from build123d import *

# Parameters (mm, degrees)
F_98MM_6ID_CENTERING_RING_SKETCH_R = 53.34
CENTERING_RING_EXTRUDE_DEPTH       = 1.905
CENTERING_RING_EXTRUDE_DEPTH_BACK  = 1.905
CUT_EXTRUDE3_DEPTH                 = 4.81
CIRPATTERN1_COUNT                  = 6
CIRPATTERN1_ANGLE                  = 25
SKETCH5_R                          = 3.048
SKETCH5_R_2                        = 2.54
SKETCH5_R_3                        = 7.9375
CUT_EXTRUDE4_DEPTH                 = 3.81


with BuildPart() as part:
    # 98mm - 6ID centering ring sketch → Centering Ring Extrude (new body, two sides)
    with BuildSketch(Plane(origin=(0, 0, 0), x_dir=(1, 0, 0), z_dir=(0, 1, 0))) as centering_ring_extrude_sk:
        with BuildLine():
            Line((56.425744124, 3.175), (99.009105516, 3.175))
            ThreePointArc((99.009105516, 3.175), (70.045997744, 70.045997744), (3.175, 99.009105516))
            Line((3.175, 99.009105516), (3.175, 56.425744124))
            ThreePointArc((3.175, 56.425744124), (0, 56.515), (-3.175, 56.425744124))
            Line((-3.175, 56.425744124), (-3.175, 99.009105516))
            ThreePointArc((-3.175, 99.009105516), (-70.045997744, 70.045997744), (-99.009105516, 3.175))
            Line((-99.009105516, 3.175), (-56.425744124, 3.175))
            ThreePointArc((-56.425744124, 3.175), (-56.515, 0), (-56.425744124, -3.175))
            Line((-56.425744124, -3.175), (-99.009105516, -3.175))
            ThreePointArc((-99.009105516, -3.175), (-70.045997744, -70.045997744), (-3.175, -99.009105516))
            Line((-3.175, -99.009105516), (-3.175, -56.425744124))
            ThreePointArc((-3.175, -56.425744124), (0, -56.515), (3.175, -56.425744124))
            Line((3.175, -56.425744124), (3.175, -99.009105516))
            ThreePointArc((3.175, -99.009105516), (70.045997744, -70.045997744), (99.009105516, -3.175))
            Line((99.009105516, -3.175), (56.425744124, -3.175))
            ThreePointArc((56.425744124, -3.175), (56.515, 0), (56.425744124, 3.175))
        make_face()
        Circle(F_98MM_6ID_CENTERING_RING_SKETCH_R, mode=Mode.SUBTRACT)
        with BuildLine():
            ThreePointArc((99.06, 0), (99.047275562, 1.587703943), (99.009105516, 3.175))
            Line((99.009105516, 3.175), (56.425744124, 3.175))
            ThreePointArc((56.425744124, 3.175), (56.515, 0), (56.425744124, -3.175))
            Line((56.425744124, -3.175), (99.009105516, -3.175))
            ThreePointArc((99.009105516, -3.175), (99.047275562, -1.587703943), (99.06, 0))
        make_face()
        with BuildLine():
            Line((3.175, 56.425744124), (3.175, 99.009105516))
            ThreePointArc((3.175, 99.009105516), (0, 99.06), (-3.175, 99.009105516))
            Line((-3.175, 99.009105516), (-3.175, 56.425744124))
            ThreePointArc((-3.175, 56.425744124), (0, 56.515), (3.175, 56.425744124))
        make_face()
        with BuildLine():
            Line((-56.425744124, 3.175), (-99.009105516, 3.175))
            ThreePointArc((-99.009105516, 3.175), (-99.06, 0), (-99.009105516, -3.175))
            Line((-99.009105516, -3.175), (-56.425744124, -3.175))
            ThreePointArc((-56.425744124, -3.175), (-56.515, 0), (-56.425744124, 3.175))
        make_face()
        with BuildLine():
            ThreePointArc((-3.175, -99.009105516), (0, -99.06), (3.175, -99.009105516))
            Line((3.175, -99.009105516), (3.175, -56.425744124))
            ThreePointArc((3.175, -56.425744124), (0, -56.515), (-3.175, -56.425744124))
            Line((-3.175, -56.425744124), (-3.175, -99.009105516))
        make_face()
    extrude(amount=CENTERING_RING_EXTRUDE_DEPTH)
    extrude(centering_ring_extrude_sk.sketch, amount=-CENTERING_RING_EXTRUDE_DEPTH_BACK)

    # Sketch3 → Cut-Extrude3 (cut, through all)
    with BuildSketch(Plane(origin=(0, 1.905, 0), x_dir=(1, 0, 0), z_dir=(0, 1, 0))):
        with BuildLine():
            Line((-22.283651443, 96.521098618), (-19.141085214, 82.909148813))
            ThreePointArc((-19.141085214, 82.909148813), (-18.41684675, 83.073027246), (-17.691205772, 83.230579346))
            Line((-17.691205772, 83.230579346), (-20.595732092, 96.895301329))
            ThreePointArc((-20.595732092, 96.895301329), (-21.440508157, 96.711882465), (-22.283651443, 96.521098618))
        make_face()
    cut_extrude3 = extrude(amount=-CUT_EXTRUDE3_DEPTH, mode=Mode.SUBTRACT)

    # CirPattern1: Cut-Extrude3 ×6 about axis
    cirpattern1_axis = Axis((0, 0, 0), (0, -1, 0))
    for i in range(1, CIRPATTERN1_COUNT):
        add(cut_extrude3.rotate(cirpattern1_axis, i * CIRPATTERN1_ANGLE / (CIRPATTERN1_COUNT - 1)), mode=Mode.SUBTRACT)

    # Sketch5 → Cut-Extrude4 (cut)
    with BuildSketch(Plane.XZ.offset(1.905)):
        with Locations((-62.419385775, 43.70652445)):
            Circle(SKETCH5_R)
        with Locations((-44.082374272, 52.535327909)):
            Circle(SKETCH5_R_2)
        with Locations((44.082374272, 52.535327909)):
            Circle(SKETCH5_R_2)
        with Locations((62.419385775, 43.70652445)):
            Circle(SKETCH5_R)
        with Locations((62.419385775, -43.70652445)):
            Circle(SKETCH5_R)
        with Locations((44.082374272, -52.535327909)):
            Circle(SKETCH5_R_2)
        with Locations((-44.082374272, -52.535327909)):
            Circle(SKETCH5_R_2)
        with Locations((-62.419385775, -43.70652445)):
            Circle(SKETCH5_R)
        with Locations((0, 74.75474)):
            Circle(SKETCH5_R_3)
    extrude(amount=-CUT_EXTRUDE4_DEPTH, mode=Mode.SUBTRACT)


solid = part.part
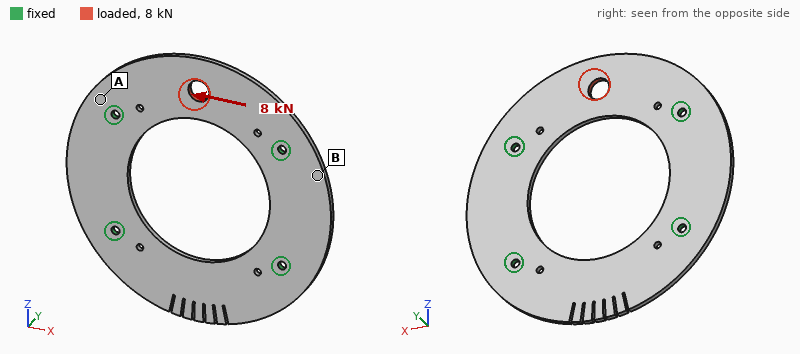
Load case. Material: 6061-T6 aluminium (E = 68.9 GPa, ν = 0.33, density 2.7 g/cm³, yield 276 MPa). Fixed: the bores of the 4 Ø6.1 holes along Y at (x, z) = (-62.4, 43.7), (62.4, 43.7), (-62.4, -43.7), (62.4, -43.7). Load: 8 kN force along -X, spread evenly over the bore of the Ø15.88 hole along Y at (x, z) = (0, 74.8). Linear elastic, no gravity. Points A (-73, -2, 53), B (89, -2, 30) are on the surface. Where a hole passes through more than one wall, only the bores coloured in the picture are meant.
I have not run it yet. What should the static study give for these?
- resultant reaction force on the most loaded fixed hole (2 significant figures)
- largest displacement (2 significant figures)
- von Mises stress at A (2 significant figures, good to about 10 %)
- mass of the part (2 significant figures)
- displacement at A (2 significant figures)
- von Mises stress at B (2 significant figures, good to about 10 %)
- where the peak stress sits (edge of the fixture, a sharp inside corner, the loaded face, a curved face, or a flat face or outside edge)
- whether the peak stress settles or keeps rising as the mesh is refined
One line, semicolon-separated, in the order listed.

4.4 kN; 53 µm; 22 MPa; 220 g; 12 µm; 9.8 MPa; edge of the fixture; keeps rising
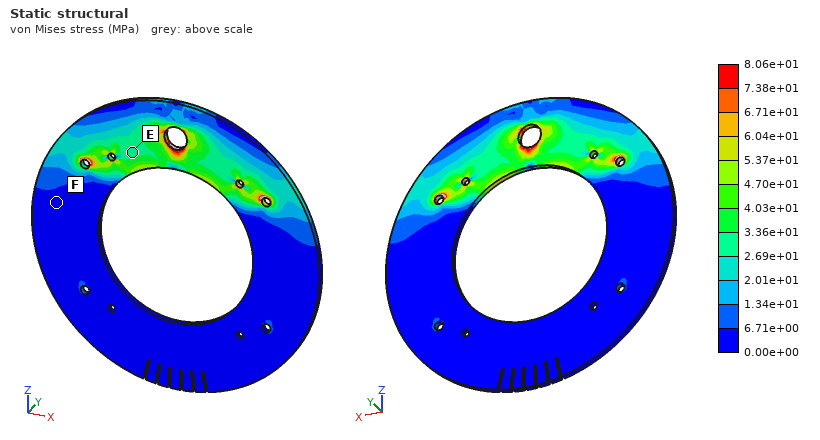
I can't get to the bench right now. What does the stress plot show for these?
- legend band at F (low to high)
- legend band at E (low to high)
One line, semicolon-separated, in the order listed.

0.00e+00 to 6.71e+00 MPa; 2.69e+01 to 3.36e+01 MPa
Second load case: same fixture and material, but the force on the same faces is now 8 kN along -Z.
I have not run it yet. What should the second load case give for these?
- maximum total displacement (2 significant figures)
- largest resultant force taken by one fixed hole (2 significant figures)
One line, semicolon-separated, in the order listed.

92 µm; 4.9 kN
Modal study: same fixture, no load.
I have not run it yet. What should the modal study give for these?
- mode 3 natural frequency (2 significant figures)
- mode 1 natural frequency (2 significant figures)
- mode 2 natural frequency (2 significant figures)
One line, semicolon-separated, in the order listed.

1700 Hz; 740 Hz; 750 Hz
